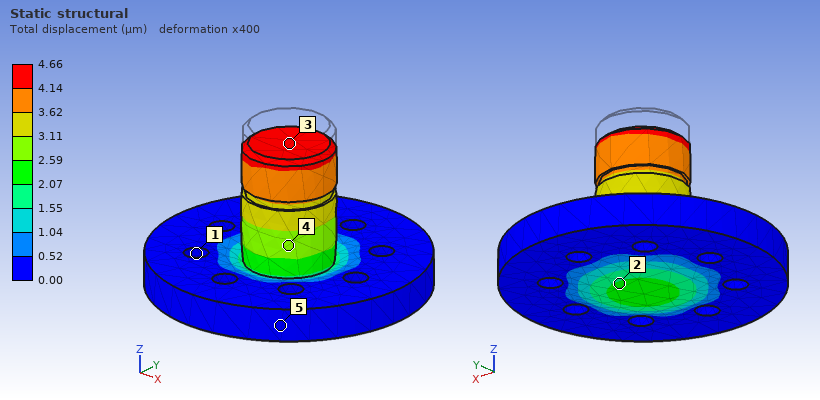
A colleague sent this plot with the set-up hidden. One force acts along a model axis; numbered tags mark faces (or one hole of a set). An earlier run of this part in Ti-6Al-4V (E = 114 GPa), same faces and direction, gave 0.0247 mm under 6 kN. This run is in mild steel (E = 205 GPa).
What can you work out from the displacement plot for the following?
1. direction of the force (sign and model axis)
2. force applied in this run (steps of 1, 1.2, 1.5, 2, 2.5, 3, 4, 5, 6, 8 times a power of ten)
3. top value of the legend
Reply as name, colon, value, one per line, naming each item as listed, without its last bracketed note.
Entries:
direction of the force: -Z
force applied in this run: 2 kN
top value of the legend: 4.66 µm
